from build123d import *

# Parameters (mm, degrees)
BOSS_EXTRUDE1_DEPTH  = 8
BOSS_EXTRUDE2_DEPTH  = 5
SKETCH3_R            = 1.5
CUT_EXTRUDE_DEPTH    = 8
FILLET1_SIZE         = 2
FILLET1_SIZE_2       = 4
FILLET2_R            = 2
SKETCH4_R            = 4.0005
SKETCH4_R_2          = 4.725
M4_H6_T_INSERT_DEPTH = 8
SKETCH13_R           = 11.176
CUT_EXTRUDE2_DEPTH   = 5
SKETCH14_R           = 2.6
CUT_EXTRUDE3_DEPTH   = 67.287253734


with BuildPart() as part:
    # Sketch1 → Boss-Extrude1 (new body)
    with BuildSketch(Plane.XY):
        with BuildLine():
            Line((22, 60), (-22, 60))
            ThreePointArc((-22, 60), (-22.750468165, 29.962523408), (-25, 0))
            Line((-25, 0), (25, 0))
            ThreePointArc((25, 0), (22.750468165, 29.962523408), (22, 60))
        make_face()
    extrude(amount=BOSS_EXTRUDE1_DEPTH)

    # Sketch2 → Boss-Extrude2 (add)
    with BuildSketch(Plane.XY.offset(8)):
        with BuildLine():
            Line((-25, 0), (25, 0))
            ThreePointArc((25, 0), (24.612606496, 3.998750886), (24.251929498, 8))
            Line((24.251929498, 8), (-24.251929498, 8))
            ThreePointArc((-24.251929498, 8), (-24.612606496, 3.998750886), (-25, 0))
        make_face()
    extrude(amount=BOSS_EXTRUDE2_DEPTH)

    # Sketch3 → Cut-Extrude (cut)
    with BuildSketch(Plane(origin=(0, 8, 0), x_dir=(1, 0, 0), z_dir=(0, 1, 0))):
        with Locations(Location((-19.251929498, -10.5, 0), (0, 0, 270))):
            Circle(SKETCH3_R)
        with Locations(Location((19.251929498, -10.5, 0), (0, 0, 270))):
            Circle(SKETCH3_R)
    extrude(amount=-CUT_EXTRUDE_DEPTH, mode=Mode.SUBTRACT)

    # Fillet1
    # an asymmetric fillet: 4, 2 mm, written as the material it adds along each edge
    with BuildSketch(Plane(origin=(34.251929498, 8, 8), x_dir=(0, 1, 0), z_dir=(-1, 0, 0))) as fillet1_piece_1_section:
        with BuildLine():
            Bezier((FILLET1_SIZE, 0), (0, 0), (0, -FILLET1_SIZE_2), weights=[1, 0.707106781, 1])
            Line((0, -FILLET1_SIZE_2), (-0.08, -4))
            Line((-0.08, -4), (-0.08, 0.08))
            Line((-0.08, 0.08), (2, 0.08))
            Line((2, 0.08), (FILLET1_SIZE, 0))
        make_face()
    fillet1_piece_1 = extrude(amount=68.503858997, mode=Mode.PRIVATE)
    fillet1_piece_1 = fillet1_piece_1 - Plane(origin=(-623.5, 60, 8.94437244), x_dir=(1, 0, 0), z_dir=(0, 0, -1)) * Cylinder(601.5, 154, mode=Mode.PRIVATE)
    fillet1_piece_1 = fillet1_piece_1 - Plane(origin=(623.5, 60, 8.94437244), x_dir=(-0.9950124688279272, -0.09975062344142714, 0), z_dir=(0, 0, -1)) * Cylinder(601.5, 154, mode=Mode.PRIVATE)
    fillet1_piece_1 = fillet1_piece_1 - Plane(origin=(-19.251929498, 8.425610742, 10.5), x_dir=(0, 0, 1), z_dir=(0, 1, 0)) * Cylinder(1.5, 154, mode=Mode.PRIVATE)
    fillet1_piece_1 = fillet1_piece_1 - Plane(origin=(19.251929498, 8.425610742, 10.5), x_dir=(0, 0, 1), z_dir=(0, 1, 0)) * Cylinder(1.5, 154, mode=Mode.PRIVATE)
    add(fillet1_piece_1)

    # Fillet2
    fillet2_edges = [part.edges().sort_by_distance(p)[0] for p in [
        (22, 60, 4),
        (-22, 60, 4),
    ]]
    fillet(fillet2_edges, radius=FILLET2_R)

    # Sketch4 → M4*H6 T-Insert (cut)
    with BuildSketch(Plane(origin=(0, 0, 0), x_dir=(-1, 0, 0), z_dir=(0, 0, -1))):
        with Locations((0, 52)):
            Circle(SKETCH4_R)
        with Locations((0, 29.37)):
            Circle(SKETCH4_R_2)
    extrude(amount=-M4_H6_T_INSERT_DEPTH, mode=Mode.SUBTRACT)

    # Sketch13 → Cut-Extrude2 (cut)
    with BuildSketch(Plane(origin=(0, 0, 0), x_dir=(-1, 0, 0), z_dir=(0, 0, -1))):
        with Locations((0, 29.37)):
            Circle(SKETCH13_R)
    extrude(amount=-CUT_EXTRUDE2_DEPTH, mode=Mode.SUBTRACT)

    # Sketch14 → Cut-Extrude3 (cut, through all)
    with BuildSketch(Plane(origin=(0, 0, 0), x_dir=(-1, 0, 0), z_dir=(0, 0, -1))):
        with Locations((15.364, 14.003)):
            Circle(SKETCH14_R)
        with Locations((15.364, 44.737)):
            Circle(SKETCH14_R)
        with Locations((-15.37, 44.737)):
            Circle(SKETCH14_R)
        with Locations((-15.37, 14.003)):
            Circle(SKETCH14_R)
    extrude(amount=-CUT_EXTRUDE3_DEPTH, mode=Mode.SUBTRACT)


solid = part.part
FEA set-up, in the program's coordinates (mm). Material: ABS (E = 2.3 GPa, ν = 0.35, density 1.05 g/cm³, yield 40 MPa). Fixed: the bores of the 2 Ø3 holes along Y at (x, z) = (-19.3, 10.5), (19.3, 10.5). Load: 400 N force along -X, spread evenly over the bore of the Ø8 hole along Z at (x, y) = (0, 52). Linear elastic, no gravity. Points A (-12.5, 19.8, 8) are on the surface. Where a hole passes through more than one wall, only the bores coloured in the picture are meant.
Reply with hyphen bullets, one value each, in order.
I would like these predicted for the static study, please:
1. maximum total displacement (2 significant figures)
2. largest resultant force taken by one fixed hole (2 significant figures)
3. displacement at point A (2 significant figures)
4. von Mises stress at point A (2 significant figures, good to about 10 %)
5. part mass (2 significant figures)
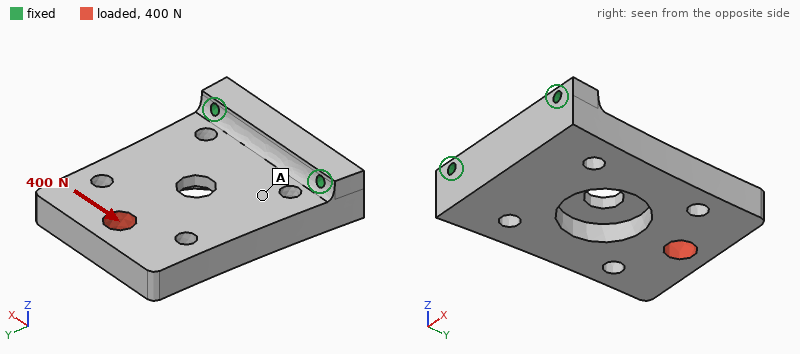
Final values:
- 0.41 mm
- 510 N
- 0.11 mm
- 2.6 MPa
- 22 g
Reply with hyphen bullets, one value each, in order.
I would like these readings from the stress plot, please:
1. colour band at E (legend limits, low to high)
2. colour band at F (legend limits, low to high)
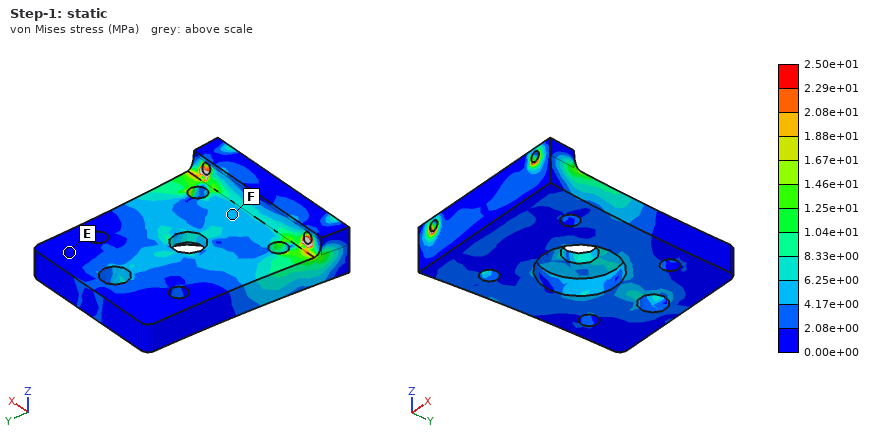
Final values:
- 0.00e+00 to 2.08e+00 MPa
- 4.17e+00 to 6.25e+00 MPa
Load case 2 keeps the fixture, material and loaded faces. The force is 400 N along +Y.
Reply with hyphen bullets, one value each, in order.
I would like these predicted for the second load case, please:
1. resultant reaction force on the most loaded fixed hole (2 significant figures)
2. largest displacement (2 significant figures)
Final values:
- 200 N
- 0.36 mm
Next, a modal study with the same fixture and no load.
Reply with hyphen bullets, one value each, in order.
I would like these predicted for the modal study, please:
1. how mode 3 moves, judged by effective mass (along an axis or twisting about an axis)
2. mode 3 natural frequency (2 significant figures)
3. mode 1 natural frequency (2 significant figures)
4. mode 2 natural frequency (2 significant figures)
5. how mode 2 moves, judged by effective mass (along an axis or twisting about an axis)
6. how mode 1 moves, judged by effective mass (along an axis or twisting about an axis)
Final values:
- along X
- 1900 Hz
- 480 Hz
- 1400 Hz
- twisting about Y
- along Z
